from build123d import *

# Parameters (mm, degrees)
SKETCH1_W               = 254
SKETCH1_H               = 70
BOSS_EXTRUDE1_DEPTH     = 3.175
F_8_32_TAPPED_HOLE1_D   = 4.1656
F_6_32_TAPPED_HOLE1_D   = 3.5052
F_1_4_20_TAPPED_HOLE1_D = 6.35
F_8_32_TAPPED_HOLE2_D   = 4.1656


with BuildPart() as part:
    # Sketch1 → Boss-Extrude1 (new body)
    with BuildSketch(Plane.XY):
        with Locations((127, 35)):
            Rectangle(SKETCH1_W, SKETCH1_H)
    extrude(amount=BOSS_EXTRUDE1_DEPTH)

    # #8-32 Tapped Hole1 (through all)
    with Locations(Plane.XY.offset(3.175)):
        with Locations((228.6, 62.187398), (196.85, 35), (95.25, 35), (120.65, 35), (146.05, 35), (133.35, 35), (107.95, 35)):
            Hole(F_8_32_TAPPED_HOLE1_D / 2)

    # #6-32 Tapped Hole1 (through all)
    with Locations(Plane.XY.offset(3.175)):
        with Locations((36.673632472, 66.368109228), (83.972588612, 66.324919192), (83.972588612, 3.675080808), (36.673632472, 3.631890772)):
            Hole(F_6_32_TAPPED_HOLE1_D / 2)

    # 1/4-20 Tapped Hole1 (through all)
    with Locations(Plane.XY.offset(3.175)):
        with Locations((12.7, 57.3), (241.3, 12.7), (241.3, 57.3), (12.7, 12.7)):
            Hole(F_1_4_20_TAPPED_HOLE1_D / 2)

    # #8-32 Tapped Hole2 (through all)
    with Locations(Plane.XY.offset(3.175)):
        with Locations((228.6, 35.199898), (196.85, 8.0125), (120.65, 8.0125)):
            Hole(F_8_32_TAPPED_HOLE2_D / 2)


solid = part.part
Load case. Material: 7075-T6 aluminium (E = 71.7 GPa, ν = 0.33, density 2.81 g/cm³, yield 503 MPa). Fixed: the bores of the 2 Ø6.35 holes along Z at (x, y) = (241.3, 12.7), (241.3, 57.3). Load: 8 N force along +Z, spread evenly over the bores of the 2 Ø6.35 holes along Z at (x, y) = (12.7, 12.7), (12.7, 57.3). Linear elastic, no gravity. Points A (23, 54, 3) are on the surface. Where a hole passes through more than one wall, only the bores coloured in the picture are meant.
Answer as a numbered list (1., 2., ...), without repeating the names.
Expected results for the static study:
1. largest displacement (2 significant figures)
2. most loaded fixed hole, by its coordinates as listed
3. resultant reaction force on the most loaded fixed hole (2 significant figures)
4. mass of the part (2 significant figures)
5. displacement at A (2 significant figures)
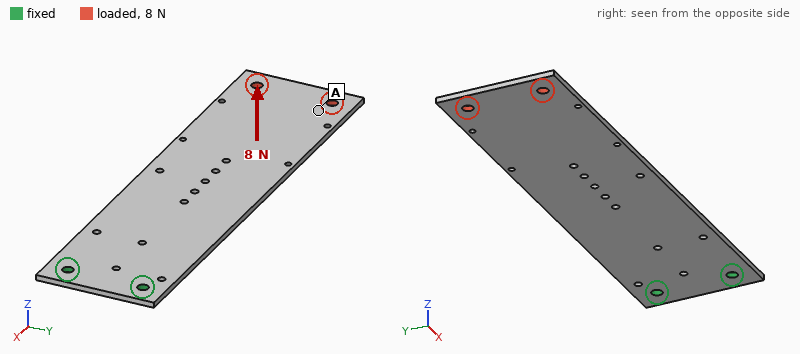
1. 2.6 mm
2. (241.3, 12.7)
3. 4.3 N
4. 160 g
5. 2.2 mm
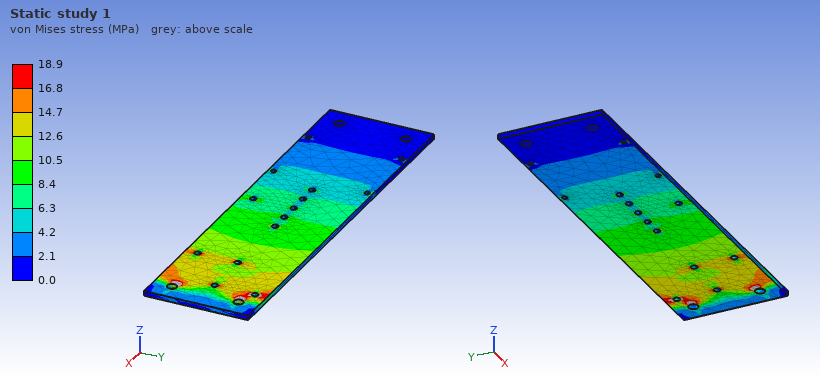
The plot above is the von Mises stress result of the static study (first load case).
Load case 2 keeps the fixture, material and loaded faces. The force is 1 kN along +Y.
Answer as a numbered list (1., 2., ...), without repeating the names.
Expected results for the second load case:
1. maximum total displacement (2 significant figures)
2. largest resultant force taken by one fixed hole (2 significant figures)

1. 0.79 mm
2. 4.9 kN
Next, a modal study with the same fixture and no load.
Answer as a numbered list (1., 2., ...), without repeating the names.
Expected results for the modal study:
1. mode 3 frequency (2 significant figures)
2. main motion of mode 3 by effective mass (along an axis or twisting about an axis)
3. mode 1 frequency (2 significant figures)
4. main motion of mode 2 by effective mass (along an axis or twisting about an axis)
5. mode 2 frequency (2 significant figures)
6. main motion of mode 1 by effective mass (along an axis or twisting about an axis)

1. 310 Hz
2. twisting about X
3. 45 Hz
4. along Z
5. 280 Hz
6. along Z
